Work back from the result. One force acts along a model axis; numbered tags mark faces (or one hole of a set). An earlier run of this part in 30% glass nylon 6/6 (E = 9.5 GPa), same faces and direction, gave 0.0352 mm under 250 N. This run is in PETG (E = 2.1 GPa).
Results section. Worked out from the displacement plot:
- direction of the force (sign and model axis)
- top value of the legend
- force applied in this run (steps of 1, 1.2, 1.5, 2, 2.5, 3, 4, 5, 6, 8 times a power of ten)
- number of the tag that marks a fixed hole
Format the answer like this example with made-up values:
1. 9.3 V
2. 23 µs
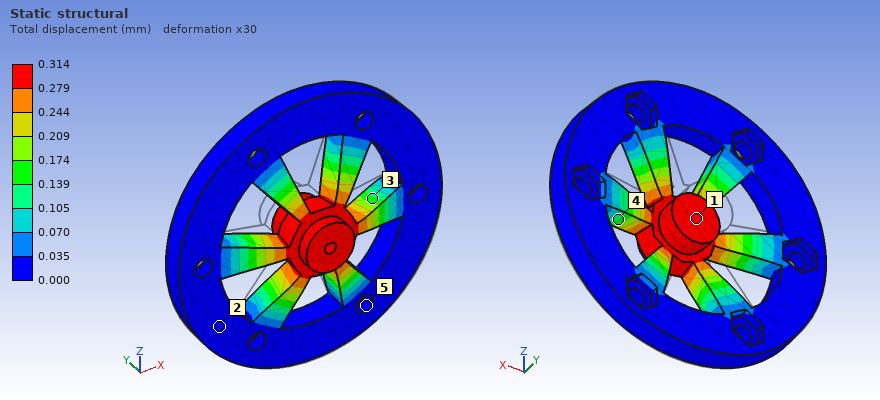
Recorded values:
1. -Y
2. 0.314 mm
3. 500 N
4. 5
